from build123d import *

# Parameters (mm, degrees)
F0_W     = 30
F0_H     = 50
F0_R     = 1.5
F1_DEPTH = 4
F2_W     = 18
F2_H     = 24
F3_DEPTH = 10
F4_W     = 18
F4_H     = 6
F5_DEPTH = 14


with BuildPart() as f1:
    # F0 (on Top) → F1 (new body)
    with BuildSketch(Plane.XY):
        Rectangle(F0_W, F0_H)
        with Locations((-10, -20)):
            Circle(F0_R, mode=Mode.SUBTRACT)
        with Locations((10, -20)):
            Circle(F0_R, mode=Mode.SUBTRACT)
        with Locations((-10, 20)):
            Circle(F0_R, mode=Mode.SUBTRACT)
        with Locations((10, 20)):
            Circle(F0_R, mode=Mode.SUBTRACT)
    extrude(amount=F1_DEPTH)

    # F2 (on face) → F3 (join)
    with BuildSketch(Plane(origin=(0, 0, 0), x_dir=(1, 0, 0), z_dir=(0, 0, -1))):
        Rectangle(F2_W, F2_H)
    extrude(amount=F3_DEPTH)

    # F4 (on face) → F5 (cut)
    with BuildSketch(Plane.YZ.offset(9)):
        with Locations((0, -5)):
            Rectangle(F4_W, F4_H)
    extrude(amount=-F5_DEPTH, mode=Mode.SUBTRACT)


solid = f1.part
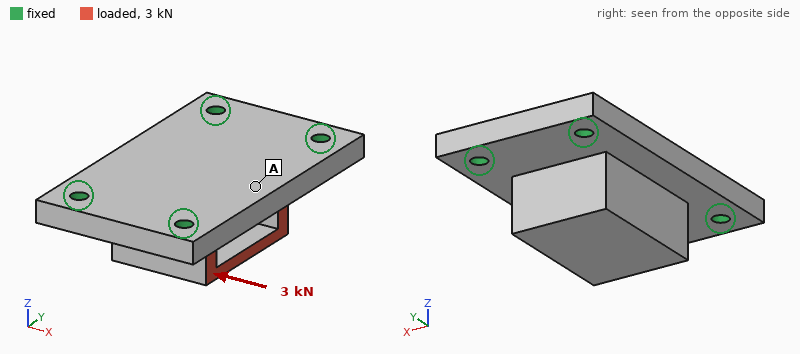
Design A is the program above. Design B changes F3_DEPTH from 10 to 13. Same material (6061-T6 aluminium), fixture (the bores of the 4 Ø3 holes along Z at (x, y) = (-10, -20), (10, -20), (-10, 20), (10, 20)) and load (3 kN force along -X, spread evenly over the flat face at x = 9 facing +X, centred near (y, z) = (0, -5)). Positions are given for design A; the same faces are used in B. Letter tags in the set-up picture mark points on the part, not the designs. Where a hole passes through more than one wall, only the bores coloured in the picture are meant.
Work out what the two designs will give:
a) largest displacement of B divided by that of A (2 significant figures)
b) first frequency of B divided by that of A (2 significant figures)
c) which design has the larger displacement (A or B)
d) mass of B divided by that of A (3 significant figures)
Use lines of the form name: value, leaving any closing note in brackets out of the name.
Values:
largest displacement of B divided by that of A: 1.4
first frequency of B divided by that of A: 0.88
which design has the larger displacement: B
mass of B divided by that of A: 1.15
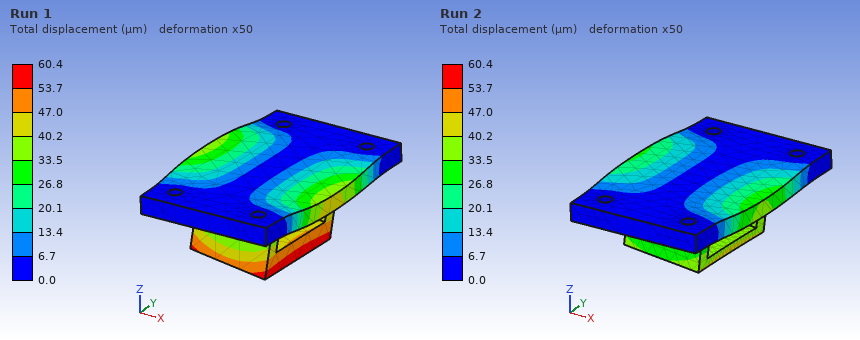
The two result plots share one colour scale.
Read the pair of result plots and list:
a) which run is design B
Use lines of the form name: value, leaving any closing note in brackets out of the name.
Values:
which run is design B: Run 1
